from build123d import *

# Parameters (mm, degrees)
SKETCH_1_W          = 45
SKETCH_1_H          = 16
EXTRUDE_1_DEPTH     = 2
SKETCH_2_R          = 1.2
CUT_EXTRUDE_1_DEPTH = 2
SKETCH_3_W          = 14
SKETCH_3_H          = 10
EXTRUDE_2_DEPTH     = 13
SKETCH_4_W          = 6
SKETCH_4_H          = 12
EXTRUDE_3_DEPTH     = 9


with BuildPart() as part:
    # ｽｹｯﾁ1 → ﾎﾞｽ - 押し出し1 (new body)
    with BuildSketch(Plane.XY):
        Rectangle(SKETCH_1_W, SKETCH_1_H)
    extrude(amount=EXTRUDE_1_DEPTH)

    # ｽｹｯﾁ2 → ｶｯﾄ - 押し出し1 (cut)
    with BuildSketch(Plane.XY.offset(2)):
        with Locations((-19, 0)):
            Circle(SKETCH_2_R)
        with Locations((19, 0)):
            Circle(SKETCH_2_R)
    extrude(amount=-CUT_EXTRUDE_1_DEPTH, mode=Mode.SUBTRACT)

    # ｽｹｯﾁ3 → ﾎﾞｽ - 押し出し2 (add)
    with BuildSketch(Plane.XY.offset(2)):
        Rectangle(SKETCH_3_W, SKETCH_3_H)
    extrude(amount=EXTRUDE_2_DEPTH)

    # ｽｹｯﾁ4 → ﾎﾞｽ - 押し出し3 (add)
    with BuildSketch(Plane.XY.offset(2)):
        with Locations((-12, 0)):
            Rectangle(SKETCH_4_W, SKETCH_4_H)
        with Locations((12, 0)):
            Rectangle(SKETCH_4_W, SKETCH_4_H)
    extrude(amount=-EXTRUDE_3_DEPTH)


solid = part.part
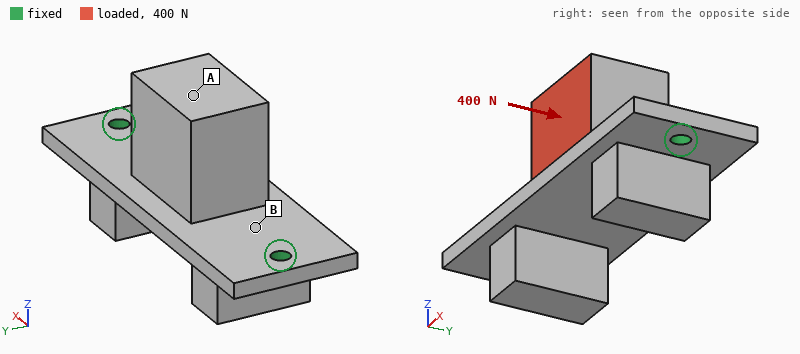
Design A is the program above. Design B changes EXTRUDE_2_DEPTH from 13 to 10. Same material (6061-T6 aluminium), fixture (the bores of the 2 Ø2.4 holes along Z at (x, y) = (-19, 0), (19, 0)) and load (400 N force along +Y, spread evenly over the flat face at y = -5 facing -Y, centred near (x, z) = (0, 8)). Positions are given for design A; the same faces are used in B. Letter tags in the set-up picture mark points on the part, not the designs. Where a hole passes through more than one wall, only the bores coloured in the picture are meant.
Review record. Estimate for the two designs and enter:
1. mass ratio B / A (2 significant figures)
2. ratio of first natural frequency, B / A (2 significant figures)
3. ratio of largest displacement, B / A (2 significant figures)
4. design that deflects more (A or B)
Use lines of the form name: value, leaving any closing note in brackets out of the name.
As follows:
mass ratio B / A: 0.90
ratio of first natural frequency, B / A: 1.2
ratio of largest displacement, B / A: 0.68
design that deflects more: A
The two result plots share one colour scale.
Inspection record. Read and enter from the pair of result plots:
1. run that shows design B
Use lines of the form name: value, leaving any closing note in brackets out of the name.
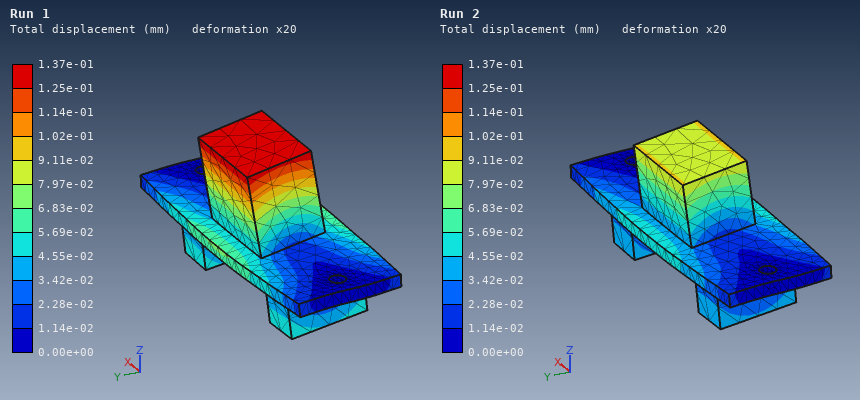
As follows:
run that shows design B: Run 2
